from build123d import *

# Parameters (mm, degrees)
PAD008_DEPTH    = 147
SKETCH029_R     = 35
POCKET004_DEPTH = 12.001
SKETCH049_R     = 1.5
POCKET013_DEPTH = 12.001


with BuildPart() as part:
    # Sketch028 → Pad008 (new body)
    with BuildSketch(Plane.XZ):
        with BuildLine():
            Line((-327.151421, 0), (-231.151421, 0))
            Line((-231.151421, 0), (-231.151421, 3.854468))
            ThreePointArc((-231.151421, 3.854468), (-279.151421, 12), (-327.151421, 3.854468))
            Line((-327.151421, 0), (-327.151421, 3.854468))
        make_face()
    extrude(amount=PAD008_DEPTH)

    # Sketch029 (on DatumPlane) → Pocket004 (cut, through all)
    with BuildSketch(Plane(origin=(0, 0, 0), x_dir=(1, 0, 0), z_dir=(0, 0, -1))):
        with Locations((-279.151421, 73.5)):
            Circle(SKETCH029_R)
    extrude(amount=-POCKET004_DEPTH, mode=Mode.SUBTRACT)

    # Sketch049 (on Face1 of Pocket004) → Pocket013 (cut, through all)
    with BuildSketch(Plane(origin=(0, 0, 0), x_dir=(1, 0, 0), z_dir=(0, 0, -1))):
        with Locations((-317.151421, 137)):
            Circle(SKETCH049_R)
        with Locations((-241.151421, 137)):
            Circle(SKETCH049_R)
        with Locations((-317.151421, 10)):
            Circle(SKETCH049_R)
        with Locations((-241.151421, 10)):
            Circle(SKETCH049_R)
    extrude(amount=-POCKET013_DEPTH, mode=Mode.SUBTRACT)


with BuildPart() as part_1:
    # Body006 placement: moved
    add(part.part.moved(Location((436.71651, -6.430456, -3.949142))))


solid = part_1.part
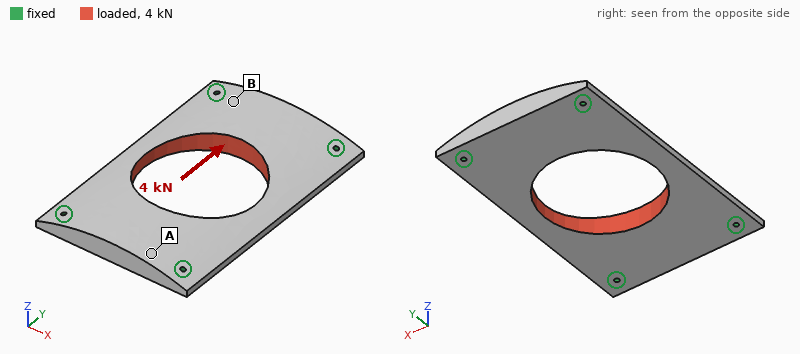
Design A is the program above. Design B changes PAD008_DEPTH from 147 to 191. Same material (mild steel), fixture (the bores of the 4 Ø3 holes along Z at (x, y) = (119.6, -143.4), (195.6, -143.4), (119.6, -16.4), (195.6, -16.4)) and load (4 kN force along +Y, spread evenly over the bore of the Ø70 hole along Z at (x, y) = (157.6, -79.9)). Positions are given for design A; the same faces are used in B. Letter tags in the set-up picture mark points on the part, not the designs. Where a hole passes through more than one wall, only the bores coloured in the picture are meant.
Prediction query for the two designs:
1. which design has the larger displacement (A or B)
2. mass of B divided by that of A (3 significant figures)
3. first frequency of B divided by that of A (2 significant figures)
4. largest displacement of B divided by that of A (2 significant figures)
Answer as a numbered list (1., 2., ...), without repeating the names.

1. B
2. 1.44
3. 0.67
4. 1.3
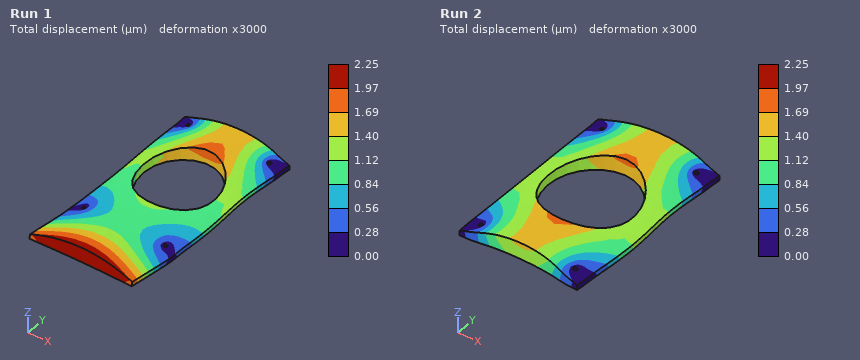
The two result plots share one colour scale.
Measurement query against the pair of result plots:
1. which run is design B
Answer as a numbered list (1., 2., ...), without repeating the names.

1. Run 1
